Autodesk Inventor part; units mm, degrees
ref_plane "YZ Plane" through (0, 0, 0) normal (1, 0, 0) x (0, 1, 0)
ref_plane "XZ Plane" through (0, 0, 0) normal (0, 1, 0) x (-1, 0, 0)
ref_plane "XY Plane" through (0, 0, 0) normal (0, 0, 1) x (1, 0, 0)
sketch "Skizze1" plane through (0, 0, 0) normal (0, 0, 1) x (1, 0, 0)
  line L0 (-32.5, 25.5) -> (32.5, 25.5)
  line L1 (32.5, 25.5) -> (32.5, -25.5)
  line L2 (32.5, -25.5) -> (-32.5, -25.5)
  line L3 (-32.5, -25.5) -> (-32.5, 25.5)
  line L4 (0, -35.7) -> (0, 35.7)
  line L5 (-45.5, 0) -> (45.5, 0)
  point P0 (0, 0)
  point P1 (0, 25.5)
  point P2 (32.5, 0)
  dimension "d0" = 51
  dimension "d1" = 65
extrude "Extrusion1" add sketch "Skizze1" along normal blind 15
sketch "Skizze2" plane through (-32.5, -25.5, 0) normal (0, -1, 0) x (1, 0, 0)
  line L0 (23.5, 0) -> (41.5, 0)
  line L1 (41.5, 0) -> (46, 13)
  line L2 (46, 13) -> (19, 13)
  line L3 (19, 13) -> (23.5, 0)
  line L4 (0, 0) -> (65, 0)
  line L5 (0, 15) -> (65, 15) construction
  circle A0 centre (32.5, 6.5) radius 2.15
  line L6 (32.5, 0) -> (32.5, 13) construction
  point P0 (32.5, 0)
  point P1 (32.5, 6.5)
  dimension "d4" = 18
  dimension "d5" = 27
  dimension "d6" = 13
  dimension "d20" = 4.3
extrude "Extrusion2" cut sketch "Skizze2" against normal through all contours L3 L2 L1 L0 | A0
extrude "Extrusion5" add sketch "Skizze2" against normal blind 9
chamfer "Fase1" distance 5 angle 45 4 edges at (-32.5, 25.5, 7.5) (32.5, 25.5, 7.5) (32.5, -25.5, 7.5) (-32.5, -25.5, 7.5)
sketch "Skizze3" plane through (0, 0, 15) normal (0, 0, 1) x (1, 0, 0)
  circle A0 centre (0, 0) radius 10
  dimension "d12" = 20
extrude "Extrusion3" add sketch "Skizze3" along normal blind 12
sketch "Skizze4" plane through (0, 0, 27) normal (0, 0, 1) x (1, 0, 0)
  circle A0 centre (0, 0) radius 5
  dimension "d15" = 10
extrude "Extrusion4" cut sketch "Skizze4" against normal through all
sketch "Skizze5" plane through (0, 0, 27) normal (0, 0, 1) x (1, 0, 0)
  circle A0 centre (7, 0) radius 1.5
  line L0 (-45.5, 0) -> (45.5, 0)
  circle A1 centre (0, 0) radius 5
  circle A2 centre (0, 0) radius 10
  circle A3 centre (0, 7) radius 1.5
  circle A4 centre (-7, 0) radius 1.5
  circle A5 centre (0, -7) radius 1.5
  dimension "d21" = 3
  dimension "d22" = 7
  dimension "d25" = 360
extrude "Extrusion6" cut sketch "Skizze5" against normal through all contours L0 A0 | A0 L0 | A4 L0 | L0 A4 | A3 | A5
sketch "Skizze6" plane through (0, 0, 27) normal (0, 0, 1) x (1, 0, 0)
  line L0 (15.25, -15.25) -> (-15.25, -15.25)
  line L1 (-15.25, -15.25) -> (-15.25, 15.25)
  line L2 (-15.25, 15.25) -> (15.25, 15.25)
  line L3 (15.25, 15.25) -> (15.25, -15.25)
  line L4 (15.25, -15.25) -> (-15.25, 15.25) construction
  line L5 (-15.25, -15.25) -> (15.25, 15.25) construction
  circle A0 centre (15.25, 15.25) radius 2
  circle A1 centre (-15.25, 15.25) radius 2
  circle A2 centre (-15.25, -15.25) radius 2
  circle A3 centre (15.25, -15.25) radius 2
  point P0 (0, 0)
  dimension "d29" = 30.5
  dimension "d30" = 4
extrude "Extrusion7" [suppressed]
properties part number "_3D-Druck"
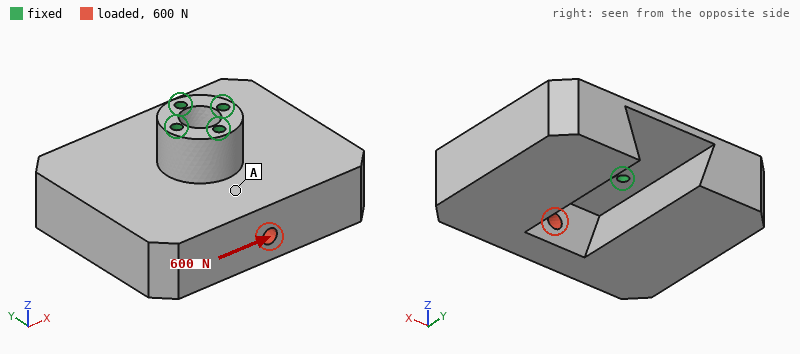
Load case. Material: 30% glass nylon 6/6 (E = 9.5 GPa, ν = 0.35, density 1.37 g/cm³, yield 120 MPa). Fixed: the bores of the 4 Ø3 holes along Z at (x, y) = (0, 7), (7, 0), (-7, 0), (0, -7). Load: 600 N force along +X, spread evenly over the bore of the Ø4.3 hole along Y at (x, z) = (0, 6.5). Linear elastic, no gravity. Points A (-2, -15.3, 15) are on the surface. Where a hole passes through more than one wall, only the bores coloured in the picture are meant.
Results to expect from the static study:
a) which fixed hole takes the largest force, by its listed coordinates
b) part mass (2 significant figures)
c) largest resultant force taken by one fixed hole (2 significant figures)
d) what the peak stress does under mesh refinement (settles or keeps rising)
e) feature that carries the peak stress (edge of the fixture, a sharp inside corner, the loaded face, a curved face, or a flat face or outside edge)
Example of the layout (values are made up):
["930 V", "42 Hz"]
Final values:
["(0, -7)", "53 g", "610 N", "keeps rising", "edge of the fixture"]
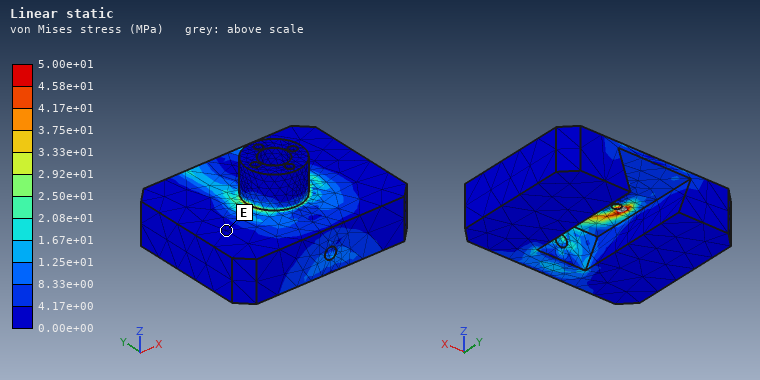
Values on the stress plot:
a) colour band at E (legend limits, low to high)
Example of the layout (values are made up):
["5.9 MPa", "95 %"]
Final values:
["0.00e+00 to 4.17e+00 MPa"]
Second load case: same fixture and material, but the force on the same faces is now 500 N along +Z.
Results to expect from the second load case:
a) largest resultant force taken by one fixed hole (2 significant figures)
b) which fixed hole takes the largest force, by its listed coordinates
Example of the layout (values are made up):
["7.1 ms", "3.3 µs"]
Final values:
["490 N", "(0, -7)"]
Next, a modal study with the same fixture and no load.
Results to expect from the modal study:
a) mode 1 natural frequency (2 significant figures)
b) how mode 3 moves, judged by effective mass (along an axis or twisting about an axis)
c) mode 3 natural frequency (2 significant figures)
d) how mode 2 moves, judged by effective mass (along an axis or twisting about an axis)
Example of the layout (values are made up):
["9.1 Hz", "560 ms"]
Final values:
["820 Hz", "along Z", "2000 Hz", "along Y"]
